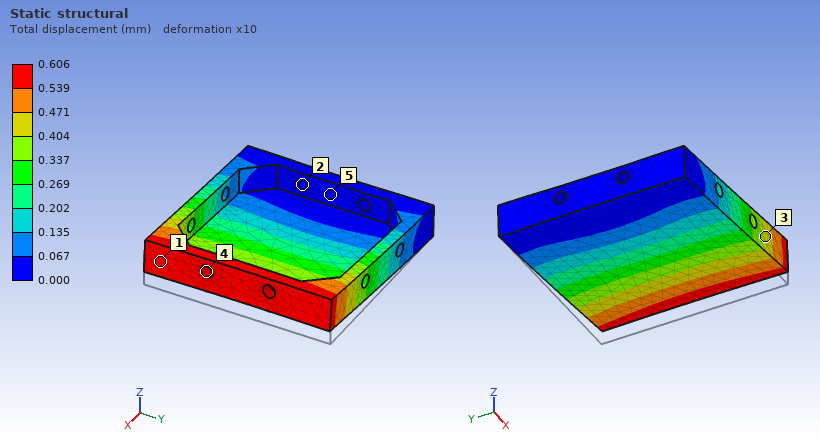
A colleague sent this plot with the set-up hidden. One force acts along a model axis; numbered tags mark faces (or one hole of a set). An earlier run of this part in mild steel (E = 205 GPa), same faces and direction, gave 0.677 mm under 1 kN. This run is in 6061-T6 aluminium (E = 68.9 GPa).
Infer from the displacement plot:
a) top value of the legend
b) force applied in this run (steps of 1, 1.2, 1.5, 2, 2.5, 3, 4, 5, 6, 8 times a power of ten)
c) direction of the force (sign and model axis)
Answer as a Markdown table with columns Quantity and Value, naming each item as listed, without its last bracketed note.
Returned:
| Quantity | Value |
|---|---|
| top value of the legend | 0.606 mm |
| force applied in this run | 300 N |
| direction of the force | +Z |
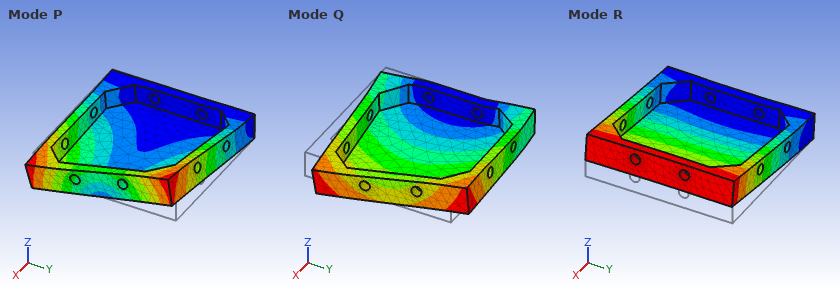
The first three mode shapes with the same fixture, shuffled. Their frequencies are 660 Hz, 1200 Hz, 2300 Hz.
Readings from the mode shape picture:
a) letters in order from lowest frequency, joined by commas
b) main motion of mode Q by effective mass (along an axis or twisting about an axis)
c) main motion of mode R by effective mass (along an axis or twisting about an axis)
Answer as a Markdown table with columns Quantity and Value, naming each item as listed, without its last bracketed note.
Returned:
| Quantity | Value |
|---|---|
| letters in order from lowest frequency, joined by commas | R, P, Q |
| main motion of mode Q by effective mass | along Y |
| main motion of mode R by effective mass | along Z |
